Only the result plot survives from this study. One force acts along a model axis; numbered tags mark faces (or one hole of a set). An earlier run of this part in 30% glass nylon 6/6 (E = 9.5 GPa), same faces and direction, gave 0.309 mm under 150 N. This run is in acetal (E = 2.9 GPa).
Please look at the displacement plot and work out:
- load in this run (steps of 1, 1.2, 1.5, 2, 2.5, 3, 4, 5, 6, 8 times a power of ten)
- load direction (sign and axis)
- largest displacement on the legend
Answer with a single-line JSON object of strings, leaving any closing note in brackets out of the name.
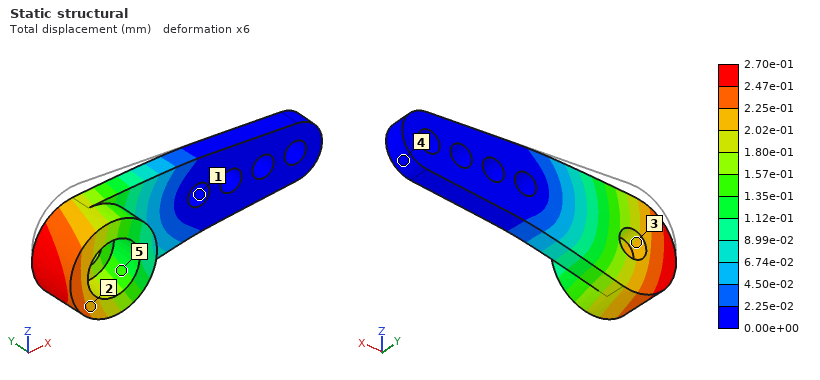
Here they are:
{"load in this run": "40 N", "load direction": "-Z", "largest displacement on the legend": "2.70e-01 mm"}
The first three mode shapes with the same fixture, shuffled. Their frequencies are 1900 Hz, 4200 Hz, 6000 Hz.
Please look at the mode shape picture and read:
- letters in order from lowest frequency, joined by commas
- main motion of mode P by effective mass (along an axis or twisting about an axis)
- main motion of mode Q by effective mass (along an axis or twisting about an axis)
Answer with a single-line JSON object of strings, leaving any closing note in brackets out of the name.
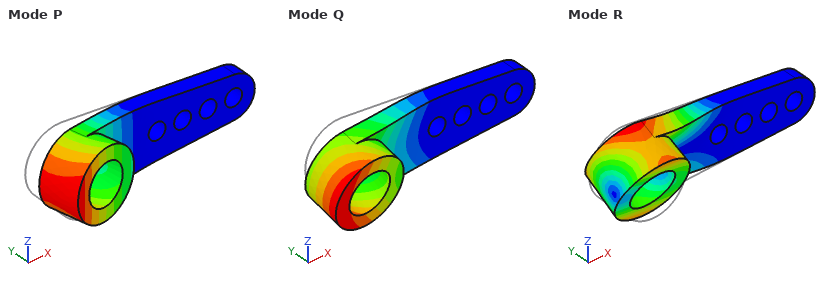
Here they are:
{"letters in order from lowest frequency, joined by commas": "P, Q, R", "main motion of mode P by effective mass": "along Y", "main motion of mode Q by effective mass": "along Z"}
